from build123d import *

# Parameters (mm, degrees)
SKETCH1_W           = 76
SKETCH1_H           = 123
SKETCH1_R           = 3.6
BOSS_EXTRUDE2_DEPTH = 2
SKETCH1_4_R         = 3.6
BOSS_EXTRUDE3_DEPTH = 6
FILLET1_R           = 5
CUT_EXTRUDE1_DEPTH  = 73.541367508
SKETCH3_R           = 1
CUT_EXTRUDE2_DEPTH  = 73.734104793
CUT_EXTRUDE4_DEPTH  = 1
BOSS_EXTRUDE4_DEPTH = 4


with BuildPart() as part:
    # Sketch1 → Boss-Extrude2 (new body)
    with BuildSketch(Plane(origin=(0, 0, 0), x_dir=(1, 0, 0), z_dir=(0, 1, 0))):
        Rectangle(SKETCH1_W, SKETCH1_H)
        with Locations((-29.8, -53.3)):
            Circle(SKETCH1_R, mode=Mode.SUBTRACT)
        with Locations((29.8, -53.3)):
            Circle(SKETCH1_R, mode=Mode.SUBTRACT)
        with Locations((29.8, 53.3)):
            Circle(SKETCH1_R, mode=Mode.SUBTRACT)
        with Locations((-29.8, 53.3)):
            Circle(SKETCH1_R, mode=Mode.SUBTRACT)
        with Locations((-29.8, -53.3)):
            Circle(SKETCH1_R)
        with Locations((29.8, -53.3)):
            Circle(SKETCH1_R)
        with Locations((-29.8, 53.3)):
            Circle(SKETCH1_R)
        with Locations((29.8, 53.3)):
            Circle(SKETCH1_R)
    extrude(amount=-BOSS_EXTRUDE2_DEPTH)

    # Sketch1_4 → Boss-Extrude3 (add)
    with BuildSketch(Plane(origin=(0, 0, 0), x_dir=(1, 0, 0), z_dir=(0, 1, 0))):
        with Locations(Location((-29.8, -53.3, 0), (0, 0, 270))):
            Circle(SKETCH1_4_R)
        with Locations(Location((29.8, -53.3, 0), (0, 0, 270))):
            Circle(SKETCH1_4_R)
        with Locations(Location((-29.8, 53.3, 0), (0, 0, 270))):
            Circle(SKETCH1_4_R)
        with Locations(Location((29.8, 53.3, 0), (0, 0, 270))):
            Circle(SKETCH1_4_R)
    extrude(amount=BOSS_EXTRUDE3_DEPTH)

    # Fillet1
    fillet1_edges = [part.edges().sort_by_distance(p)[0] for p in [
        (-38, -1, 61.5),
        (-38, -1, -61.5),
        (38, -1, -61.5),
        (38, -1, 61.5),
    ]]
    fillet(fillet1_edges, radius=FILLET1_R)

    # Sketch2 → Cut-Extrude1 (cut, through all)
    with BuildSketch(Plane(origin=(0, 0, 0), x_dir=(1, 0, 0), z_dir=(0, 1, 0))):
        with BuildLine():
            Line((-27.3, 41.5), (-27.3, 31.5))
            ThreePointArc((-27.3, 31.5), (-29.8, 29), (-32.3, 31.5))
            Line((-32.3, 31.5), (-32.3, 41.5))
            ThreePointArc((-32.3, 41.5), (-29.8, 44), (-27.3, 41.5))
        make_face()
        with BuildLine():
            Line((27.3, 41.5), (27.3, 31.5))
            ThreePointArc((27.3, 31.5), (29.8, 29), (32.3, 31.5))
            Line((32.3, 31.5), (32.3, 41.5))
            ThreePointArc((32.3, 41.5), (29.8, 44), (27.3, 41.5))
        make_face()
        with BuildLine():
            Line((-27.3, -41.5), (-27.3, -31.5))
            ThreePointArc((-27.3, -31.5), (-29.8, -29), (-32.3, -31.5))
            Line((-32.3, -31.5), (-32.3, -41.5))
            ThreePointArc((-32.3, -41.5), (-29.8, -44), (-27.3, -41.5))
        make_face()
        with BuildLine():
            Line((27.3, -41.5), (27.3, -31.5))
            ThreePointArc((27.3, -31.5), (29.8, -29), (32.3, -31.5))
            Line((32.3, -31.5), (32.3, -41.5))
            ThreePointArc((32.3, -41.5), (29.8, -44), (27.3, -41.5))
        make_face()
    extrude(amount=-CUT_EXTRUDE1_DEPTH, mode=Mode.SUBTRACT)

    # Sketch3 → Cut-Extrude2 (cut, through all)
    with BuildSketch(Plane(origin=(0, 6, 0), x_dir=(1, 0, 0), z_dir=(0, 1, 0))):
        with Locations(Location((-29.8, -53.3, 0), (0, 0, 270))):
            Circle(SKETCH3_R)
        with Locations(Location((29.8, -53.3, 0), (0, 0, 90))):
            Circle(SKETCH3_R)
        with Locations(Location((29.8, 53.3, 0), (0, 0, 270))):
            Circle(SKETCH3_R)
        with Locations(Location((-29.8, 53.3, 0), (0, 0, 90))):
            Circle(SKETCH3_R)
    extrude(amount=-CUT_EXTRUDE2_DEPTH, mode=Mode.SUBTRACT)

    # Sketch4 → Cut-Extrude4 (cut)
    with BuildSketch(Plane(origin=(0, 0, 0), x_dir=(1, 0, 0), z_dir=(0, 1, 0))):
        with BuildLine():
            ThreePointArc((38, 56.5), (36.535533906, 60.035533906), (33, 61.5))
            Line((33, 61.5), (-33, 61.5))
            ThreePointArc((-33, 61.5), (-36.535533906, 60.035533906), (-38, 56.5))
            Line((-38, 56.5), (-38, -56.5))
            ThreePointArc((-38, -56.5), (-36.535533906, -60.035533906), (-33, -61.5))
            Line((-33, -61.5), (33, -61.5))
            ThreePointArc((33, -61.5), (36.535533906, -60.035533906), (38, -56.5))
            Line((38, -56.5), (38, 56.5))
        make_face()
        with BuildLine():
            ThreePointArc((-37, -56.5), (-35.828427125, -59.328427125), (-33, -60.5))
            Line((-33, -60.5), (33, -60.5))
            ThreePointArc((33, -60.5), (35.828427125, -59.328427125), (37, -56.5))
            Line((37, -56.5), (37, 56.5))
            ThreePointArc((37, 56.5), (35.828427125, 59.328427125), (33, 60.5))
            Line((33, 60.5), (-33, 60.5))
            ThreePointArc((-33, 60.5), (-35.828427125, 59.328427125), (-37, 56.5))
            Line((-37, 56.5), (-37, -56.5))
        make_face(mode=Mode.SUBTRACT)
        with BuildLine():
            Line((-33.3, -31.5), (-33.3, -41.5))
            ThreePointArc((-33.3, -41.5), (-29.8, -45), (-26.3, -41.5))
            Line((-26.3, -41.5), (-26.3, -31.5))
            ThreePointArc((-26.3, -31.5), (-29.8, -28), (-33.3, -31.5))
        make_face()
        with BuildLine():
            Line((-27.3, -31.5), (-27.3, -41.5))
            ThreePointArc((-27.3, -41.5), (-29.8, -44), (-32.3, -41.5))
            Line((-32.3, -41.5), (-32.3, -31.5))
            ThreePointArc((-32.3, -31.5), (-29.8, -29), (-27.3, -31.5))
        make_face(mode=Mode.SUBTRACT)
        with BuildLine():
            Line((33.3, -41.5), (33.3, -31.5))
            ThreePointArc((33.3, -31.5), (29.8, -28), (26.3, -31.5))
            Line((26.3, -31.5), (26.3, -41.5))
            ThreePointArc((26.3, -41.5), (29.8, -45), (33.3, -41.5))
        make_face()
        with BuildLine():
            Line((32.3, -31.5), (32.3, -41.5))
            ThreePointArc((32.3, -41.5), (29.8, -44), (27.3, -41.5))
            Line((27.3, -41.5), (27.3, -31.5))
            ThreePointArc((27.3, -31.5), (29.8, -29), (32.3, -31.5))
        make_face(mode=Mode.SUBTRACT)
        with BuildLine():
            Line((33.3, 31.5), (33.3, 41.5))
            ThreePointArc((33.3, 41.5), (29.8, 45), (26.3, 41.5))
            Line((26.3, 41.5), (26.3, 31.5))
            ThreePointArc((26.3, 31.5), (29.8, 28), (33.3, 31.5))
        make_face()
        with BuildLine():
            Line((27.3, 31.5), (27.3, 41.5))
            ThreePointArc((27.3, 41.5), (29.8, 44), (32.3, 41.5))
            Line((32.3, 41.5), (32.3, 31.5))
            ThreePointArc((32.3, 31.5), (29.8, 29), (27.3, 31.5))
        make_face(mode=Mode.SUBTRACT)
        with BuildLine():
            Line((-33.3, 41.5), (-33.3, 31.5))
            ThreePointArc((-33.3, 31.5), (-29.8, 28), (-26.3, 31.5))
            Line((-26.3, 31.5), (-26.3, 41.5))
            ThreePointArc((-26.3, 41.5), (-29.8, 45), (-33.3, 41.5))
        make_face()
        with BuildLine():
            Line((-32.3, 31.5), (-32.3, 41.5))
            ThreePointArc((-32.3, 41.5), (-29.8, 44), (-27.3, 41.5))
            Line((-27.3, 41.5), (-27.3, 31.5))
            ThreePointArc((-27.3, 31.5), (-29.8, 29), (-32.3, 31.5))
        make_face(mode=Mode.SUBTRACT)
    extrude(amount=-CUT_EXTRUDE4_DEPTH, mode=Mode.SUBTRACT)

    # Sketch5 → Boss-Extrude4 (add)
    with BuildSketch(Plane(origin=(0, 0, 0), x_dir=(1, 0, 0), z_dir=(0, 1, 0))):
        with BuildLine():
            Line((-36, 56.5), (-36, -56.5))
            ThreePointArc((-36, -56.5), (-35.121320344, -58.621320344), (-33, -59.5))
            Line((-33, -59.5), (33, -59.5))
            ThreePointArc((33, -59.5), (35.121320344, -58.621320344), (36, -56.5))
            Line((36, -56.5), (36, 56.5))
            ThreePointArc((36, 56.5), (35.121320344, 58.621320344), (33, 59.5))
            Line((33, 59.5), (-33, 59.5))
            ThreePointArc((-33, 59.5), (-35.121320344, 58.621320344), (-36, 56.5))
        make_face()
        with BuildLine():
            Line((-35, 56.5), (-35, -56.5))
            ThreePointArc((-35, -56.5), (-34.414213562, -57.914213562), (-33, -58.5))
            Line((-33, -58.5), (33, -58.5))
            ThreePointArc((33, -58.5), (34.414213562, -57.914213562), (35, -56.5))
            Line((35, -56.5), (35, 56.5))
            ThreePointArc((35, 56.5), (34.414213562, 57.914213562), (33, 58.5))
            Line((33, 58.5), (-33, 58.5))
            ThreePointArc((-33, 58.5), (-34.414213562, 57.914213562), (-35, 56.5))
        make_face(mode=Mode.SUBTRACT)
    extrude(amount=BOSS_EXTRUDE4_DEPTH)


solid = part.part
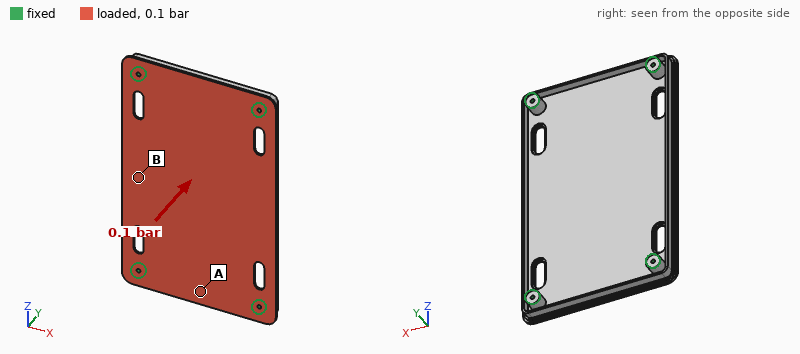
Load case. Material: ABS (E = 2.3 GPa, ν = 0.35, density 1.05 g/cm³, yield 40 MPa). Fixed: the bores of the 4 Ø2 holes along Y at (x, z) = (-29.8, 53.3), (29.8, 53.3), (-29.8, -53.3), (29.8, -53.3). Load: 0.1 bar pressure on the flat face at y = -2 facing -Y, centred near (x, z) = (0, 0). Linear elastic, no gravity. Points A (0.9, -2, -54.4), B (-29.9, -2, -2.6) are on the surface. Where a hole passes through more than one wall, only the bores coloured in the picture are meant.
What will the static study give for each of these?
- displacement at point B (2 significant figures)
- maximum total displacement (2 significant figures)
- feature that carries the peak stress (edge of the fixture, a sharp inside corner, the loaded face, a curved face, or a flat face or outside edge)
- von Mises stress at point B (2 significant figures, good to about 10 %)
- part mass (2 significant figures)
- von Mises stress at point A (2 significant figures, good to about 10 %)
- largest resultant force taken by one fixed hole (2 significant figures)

1.2 mm
1.7 mm
the loaded face
4.0 MPa
21 g
2.1 MPa
24 N
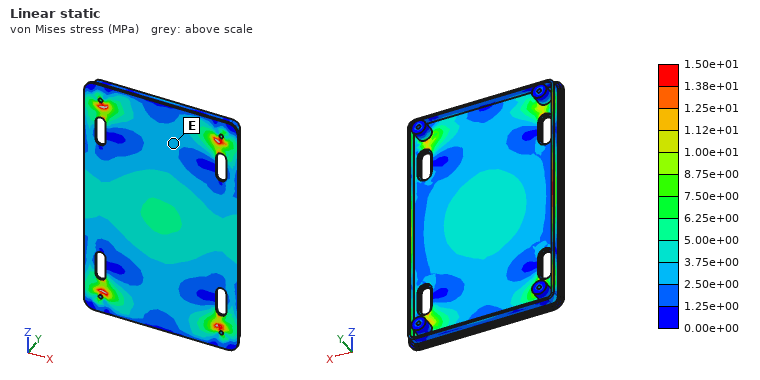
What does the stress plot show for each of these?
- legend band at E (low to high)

2.50e+00 to 3.75e+00 MPa
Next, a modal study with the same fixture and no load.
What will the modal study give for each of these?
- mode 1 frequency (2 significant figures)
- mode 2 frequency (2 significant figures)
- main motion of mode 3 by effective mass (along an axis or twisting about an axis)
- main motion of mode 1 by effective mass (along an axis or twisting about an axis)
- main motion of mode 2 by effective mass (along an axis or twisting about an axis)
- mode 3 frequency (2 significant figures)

320 Hz
510 Hz
twisting about X
along Y
twisting about Z
740 Hz
